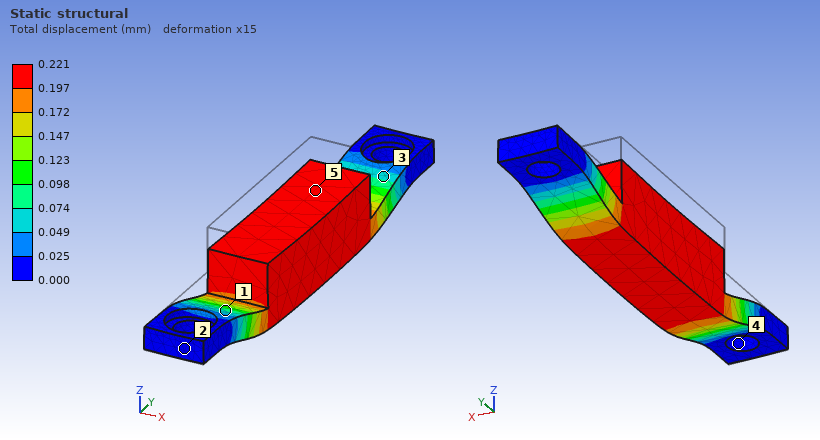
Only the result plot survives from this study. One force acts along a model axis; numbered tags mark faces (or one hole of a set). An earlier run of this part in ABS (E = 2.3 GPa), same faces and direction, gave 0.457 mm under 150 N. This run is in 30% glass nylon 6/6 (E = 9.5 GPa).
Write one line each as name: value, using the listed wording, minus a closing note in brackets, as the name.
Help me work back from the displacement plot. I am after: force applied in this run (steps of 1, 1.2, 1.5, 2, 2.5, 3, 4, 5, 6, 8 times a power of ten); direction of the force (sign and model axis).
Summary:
force applied in this run: 300 N
direction of the force: -Z
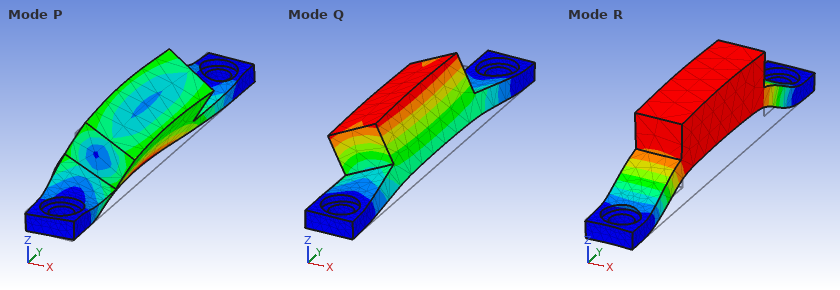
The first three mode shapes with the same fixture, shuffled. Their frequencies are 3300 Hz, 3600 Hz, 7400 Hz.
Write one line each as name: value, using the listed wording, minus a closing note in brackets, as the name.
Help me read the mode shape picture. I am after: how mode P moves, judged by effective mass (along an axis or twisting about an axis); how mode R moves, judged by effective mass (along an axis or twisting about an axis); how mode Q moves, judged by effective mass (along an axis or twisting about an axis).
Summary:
how mode P moves, judged by effective mass: along X
how mode R moves, judged by effective mass: along Z
how mode Q moves, judged by effective mass: along X
